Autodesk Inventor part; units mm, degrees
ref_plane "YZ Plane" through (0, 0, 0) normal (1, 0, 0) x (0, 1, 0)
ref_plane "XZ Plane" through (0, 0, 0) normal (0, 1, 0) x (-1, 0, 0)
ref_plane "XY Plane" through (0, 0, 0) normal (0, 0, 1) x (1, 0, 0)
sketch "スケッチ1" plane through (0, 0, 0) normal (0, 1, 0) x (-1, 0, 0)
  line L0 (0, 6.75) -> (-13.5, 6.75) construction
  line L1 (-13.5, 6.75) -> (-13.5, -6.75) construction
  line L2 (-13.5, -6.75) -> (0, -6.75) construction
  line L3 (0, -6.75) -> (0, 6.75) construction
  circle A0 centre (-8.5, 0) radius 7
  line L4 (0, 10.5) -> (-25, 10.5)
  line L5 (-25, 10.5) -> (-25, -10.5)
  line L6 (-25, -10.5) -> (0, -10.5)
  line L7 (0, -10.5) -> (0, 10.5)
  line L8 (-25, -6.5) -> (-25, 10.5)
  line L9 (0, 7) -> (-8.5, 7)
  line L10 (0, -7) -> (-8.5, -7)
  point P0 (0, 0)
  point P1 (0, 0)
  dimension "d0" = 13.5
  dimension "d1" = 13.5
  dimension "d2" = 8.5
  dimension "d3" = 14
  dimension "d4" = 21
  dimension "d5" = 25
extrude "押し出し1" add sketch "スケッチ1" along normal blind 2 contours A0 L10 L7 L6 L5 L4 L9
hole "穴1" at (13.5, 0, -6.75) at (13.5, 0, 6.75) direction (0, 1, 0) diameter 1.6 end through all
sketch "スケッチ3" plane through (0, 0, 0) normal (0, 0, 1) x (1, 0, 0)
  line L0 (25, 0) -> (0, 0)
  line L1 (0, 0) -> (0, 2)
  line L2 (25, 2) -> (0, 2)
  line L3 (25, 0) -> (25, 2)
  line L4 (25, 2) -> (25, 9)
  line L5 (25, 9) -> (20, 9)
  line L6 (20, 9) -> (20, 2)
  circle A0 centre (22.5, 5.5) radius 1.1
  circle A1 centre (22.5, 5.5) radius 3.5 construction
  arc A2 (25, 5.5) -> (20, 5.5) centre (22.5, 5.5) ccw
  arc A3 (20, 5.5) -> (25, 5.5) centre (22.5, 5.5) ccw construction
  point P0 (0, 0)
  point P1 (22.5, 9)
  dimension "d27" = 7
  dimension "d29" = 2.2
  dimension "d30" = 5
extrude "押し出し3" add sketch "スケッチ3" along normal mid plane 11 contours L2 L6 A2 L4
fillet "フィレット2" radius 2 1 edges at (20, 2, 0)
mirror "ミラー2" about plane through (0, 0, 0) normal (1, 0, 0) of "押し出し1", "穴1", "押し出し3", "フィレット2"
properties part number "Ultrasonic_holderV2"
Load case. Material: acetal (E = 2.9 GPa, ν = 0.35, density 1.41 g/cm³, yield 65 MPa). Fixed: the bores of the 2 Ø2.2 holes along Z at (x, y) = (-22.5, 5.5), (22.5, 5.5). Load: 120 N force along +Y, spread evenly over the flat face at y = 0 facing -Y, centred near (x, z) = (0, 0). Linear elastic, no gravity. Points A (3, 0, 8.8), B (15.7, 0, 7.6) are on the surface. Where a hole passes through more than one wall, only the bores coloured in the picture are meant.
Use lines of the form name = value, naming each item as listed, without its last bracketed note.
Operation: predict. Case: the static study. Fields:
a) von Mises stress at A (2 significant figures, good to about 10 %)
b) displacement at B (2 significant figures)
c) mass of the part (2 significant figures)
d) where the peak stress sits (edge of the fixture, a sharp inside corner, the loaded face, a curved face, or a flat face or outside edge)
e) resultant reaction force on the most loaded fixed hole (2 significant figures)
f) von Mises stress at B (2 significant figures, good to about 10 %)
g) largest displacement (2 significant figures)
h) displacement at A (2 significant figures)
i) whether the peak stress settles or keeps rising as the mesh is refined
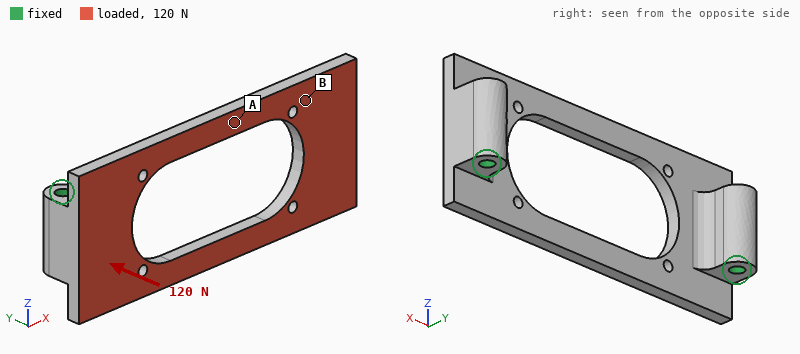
von Mises stress at A = 16 MPa
displacement at B = 0.13 mm
mass of the part = 2.6 g
where the peak stress sits = a sharp inside corner
resultant reaction force on the most loaded fixed hole = 63 N
von Mises stress at B = 9.2 MPa
largest displacement = 0.62 mm
displacement at A = 0.56 mm
whether the peak stress settles or keeps rising as the mesh is refined = keeps rising
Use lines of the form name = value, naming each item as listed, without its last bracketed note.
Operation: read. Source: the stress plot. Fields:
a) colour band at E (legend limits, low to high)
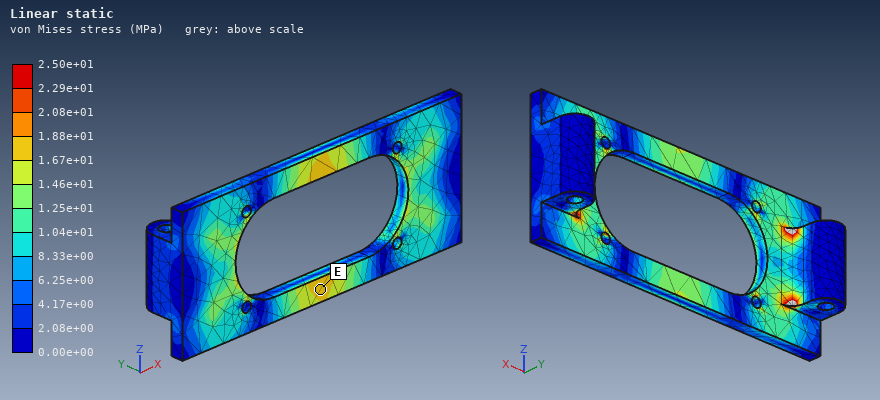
colour band at E = 1.67e+01 to 1.88e+01 MPa
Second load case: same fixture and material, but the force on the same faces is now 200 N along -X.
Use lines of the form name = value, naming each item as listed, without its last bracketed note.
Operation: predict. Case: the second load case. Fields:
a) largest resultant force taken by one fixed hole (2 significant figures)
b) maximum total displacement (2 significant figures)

largest resultant force taken by one fixed hole = 100 N
maximum total displacement = 59 µm
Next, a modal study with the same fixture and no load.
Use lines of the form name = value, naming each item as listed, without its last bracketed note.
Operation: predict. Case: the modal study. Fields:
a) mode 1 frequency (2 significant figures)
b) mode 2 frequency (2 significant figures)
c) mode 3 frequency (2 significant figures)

mode 1 frequency = 2000 Hz
mode 2 frequency = 2000 Hz
mode 3 frequency = 4500 Hz
